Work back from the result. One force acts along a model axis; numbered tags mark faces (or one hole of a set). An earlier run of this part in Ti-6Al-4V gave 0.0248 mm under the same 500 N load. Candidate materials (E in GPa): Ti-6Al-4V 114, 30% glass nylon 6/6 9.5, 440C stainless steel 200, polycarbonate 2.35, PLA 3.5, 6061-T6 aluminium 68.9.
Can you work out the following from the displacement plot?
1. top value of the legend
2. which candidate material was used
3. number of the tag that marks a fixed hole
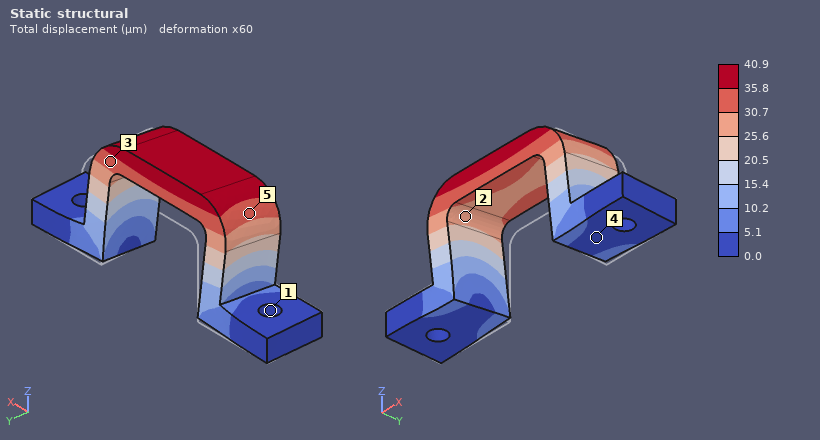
40.9 µm
6061-T6 aluminium
1
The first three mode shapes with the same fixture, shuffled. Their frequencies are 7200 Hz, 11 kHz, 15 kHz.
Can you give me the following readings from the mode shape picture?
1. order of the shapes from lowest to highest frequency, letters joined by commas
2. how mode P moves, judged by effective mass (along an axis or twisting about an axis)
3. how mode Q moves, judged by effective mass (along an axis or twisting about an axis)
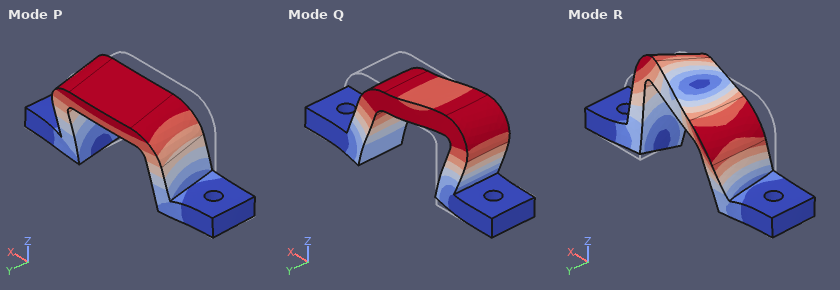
P, Q, R
along Y
along X
